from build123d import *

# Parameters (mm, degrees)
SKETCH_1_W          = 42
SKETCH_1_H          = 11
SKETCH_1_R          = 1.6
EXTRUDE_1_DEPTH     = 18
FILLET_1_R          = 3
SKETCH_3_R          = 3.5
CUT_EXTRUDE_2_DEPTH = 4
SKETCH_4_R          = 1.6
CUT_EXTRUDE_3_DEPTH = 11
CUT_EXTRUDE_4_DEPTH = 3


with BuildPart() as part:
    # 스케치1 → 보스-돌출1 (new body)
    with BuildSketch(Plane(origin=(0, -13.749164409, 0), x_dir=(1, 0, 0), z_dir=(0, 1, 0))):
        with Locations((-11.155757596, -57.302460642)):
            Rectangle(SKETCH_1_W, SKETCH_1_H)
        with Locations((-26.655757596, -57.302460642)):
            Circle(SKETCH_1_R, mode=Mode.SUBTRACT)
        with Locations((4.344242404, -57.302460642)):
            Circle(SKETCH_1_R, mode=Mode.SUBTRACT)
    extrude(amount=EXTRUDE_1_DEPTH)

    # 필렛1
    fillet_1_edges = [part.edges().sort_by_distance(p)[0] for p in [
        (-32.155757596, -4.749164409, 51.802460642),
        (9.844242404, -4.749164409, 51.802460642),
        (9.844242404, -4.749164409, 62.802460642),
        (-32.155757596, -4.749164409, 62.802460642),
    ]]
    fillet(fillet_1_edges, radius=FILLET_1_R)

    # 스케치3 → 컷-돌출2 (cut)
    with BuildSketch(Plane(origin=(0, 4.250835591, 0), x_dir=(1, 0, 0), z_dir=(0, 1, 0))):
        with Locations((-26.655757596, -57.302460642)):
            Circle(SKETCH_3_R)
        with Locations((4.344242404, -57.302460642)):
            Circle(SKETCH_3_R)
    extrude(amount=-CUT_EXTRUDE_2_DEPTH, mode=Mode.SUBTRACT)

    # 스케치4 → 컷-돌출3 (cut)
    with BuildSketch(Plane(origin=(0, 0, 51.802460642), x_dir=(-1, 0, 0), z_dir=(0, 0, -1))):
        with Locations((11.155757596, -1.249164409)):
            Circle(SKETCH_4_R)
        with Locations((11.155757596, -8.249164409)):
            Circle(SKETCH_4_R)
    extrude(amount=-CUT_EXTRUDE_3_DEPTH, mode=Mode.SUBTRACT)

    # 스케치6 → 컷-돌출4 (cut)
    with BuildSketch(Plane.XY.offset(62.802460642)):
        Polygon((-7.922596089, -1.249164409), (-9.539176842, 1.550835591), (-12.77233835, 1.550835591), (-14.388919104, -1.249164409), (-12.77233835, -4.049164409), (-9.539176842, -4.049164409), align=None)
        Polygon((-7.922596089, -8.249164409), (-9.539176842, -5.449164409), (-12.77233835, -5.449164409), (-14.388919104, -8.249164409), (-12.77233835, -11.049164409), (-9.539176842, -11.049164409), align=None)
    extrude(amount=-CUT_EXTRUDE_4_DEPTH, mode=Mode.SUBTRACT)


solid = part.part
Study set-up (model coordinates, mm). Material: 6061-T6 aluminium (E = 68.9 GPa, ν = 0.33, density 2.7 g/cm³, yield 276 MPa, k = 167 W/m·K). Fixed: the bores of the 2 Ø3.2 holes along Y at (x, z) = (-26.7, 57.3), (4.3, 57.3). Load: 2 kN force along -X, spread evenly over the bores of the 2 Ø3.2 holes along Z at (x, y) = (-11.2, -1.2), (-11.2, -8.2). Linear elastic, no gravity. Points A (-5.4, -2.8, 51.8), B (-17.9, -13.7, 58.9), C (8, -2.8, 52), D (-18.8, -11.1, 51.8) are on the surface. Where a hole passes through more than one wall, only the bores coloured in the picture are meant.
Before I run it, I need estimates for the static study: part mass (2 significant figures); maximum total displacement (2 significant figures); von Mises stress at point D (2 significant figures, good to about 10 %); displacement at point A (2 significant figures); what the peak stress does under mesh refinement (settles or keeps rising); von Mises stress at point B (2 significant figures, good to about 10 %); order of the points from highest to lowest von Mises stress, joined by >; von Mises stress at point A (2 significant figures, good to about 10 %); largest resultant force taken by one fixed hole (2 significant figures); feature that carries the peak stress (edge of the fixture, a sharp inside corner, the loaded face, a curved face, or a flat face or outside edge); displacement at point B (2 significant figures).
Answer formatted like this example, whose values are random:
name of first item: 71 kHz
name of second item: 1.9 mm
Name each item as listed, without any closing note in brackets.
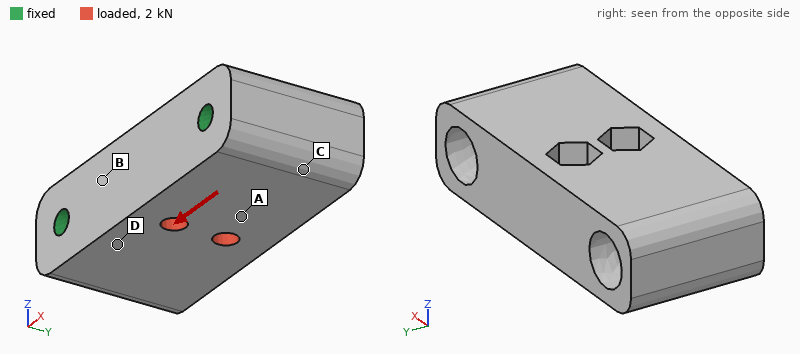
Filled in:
part mass: 20 g
maximum total displacement: 2.0 µm
von Mises stress at point D: 6.5 MPa
displacement at point A: 1.2 µm
what the peak stress does under mesh refinement: keeps rising
von Mises stress at point B: 3.9 MPa
order of the points from highest to lowest von Mises stress, joined by >: A > D > B > C
von Mises stress at point A: 9.0 MPa
largest resultant force taken by one fixed hole: 1.0 kN
feature that carries the peak stress: edge of the fixture
displacement at point B: 0.72 µm
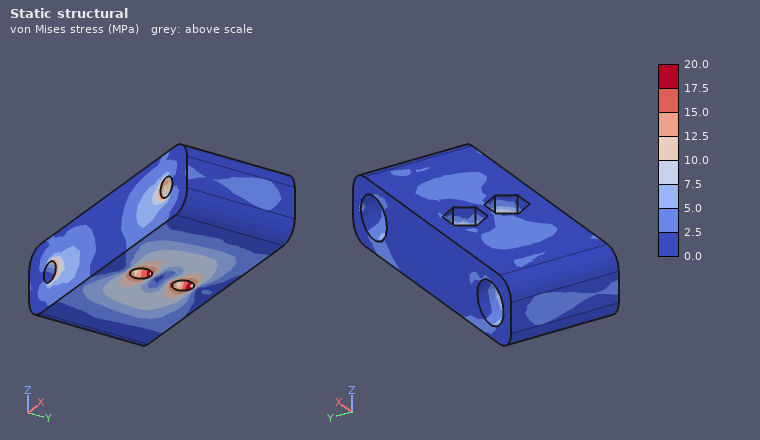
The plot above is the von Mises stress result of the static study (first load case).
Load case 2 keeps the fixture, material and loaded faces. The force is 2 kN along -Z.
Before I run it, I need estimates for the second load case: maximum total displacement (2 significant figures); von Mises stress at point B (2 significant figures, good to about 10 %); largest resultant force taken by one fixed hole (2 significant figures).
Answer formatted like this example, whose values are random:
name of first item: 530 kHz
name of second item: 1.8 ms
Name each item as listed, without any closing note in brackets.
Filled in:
maximum total displacement: 11 µm
von Mises stress at point B: 14 MPa
largest resultant force taken by one fixed hole: 1.0 kN
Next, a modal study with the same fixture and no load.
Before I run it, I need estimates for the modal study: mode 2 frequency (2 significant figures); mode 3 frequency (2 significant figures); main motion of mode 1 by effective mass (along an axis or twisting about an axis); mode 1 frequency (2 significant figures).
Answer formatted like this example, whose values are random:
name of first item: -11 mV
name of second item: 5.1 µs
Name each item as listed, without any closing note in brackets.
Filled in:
mode 2 frequency: 38 kHz
mode 3 frequency: 40 kHz
main motion of mode 1 by effective mass: along Z
mode 1 frequency: 27 kHz
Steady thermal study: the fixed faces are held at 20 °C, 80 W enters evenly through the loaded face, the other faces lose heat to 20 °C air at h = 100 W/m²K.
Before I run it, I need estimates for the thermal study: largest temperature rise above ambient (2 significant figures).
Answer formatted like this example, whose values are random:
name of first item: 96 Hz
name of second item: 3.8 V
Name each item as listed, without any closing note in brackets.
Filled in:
largest temperature rise above ambient: 24 K
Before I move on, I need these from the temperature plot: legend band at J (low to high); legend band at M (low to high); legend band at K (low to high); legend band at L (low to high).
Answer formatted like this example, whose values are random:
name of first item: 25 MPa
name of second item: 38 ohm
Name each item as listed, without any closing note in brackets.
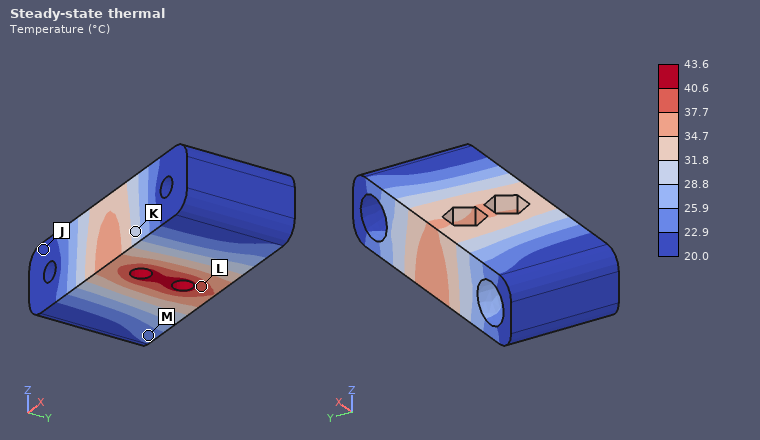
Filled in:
legend band at J: 20.0 to 22.9 °C
legend band at M: 22.9 to 25.9 °C
legend band at K: 28.8 to 31.8 °C
legend band at L: 37.7 to 40.6 °C
